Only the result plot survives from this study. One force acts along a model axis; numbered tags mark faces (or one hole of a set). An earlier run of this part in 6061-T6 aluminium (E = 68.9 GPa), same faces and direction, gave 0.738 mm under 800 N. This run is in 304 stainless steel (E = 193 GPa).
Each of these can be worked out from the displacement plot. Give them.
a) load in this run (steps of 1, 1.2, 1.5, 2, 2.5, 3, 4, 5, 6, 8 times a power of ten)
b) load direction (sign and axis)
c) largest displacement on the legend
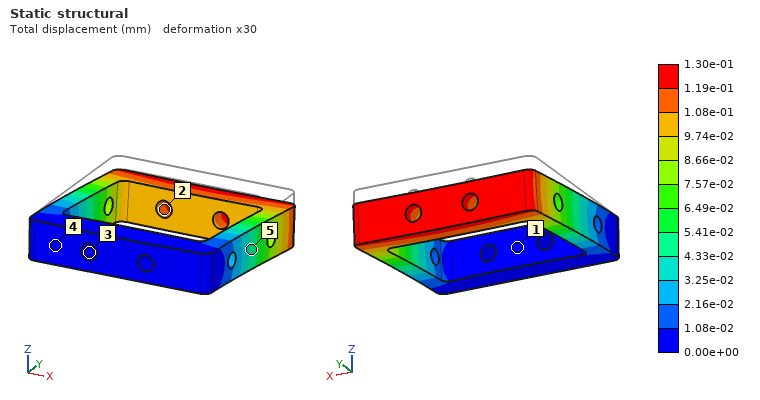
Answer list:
400 N
-Z
1.30e-01 mm
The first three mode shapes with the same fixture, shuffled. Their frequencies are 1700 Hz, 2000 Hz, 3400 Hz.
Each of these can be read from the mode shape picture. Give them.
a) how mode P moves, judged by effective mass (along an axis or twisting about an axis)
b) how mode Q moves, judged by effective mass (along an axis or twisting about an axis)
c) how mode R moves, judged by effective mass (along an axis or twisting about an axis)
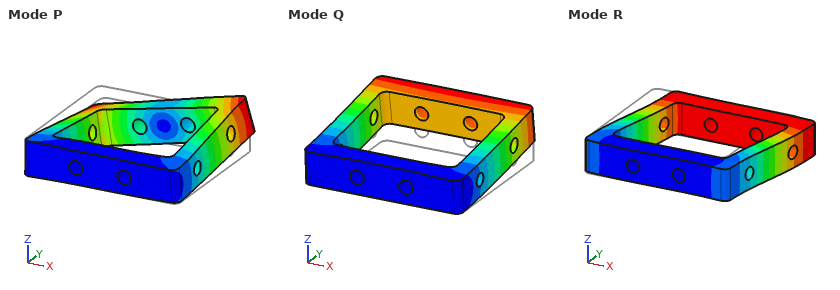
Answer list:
twisting about Y
along Z
along X
